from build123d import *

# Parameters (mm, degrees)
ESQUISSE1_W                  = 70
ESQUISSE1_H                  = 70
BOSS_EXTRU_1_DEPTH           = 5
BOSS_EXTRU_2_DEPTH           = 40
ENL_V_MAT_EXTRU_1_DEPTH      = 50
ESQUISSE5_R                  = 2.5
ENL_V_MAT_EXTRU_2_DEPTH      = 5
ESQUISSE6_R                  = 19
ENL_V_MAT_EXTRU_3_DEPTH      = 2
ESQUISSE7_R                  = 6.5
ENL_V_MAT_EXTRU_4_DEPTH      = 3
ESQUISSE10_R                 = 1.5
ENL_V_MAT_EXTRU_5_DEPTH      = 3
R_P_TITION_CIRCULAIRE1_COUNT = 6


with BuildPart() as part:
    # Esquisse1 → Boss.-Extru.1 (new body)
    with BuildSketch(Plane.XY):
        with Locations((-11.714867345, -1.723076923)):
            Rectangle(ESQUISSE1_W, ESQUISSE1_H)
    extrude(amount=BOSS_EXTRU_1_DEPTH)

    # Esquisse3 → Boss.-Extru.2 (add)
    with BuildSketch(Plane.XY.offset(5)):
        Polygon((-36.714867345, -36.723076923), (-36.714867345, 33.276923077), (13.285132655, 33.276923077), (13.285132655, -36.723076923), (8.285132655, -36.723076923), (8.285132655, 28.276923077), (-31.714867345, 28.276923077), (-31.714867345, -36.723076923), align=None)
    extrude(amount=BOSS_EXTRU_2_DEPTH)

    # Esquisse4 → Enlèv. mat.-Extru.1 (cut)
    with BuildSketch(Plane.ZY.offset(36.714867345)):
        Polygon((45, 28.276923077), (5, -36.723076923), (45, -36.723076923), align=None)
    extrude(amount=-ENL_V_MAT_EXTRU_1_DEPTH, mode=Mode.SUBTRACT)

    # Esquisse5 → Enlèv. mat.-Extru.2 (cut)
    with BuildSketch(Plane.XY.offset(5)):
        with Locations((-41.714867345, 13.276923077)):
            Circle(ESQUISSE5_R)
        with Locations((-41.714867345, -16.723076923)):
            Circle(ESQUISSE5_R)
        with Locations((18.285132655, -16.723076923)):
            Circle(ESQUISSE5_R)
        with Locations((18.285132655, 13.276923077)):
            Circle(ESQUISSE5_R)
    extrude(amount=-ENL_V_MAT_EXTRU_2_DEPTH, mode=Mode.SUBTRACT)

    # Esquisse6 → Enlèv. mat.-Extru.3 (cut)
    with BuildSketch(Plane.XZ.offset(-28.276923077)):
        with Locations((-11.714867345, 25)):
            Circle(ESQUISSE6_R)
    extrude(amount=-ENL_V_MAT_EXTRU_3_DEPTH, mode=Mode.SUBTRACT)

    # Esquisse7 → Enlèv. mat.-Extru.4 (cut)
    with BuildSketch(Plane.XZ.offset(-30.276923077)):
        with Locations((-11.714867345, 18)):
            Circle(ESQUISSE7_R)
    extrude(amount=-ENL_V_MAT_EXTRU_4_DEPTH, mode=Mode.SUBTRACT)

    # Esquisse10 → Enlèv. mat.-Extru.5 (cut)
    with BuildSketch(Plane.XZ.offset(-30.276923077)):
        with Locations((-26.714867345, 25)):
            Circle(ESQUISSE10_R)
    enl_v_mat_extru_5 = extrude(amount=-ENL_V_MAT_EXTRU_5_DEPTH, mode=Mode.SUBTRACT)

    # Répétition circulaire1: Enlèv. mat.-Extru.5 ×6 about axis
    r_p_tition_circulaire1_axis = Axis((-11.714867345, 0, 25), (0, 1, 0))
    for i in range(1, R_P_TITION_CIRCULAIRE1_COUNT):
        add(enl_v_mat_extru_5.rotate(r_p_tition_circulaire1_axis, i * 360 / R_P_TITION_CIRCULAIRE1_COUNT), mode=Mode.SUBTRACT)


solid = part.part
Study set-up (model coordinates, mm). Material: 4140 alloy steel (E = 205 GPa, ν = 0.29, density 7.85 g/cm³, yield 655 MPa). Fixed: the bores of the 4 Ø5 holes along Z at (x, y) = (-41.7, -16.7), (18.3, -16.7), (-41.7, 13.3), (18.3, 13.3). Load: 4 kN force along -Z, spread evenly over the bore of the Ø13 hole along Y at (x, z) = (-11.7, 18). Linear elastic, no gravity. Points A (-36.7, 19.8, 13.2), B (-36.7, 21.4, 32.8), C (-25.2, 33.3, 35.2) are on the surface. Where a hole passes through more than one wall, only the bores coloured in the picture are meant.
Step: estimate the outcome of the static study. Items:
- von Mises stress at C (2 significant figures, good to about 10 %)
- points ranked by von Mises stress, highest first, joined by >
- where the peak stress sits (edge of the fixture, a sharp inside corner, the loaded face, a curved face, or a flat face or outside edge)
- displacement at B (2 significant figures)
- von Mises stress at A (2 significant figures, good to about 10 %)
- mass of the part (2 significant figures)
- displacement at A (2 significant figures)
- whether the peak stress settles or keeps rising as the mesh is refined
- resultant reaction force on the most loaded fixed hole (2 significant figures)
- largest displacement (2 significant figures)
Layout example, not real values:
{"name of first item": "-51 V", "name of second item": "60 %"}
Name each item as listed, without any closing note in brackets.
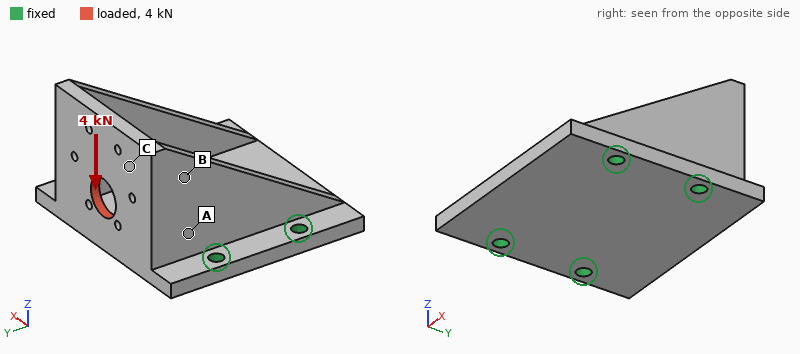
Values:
{"von Mises stress at C": "22 MPa", "points ranked by von Mises stress, highest first, joined by >": "A > C > B", "where the peak stress sits": "edge of the fixture", "displacement at B": "19 µm", "von Mises stress at A": "39 MPa", "mass of the part": "350 g", "displacement at A": "11 µm", "whether the peak stress settles or keeps rising as the mesh is refined": "keeps rising", "resultant reaction force on the most loaded fixed hole": "3.1 kN", "largest displacement": "36 µm"}
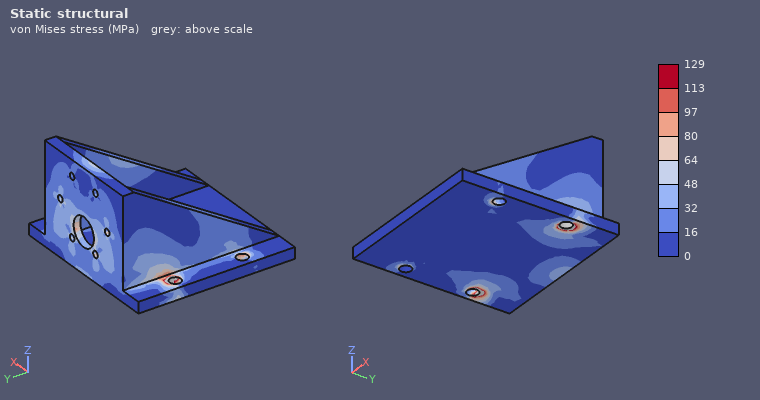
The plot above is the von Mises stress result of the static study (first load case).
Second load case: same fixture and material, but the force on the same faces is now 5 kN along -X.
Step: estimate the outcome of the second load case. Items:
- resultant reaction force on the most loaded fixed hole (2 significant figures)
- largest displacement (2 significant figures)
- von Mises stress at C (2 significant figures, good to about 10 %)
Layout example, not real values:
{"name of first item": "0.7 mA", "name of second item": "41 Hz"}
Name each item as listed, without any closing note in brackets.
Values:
{"resultant reaction force on the most loaded fixed hole": "3.3 kN", "largest displacement": "29 µm", "von Mises stress at C": "21 MPa"}
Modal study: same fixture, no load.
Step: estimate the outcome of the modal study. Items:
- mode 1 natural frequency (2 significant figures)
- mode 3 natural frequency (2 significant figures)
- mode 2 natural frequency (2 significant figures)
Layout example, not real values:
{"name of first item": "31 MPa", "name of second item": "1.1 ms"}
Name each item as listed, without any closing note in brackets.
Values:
{"mode 1 natural frequency": "5100 Hz", "mode 3 natural frequency": "5900 Hz", "mode 2 natural frequency": "5900 Hz"}
